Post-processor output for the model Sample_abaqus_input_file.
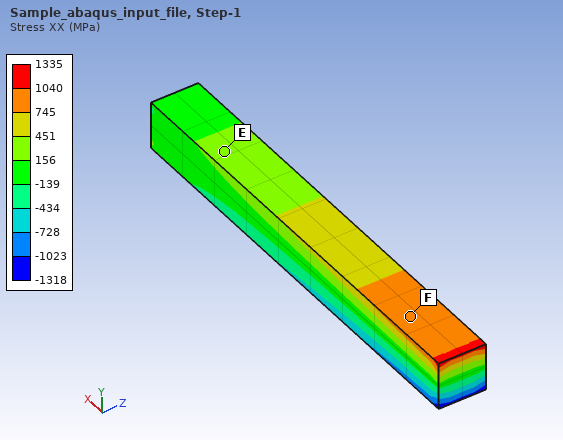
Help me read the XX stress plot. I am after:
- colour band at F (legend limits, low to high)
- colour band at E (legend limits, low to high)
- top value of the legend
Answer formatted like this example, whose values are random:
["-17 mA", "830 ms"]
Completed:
["745 to 1040 MPa", "156 to 451 MPa", "1335 MPa"]
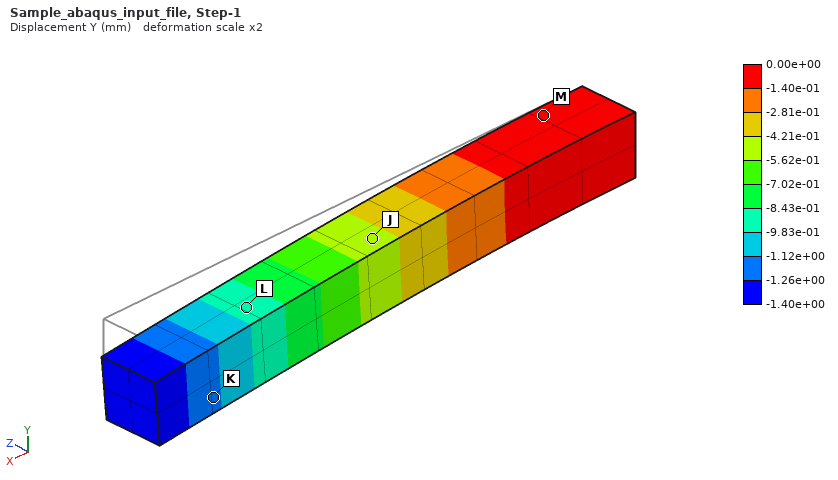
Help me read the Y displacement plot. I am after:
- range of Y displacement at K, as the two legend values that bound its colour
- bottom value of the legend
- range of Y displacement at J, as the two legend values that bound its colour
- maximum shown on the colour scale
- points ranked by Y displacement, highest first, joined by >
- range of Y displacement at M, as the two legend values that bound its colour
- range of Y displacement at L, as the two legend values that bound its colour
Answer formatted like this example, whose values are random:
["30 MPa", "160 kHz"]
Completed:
["-1.26e+00 to -1.12e+00 mm", "-1.40e+00 mm", "-5.62e-01 to -4.21e-01 mm", "0.00e+00 mm", "M > J > L > K", "-1.40e-01 to 0.00e+00 mm", "-9.83e-01 to -8.43e-01 mm"]
